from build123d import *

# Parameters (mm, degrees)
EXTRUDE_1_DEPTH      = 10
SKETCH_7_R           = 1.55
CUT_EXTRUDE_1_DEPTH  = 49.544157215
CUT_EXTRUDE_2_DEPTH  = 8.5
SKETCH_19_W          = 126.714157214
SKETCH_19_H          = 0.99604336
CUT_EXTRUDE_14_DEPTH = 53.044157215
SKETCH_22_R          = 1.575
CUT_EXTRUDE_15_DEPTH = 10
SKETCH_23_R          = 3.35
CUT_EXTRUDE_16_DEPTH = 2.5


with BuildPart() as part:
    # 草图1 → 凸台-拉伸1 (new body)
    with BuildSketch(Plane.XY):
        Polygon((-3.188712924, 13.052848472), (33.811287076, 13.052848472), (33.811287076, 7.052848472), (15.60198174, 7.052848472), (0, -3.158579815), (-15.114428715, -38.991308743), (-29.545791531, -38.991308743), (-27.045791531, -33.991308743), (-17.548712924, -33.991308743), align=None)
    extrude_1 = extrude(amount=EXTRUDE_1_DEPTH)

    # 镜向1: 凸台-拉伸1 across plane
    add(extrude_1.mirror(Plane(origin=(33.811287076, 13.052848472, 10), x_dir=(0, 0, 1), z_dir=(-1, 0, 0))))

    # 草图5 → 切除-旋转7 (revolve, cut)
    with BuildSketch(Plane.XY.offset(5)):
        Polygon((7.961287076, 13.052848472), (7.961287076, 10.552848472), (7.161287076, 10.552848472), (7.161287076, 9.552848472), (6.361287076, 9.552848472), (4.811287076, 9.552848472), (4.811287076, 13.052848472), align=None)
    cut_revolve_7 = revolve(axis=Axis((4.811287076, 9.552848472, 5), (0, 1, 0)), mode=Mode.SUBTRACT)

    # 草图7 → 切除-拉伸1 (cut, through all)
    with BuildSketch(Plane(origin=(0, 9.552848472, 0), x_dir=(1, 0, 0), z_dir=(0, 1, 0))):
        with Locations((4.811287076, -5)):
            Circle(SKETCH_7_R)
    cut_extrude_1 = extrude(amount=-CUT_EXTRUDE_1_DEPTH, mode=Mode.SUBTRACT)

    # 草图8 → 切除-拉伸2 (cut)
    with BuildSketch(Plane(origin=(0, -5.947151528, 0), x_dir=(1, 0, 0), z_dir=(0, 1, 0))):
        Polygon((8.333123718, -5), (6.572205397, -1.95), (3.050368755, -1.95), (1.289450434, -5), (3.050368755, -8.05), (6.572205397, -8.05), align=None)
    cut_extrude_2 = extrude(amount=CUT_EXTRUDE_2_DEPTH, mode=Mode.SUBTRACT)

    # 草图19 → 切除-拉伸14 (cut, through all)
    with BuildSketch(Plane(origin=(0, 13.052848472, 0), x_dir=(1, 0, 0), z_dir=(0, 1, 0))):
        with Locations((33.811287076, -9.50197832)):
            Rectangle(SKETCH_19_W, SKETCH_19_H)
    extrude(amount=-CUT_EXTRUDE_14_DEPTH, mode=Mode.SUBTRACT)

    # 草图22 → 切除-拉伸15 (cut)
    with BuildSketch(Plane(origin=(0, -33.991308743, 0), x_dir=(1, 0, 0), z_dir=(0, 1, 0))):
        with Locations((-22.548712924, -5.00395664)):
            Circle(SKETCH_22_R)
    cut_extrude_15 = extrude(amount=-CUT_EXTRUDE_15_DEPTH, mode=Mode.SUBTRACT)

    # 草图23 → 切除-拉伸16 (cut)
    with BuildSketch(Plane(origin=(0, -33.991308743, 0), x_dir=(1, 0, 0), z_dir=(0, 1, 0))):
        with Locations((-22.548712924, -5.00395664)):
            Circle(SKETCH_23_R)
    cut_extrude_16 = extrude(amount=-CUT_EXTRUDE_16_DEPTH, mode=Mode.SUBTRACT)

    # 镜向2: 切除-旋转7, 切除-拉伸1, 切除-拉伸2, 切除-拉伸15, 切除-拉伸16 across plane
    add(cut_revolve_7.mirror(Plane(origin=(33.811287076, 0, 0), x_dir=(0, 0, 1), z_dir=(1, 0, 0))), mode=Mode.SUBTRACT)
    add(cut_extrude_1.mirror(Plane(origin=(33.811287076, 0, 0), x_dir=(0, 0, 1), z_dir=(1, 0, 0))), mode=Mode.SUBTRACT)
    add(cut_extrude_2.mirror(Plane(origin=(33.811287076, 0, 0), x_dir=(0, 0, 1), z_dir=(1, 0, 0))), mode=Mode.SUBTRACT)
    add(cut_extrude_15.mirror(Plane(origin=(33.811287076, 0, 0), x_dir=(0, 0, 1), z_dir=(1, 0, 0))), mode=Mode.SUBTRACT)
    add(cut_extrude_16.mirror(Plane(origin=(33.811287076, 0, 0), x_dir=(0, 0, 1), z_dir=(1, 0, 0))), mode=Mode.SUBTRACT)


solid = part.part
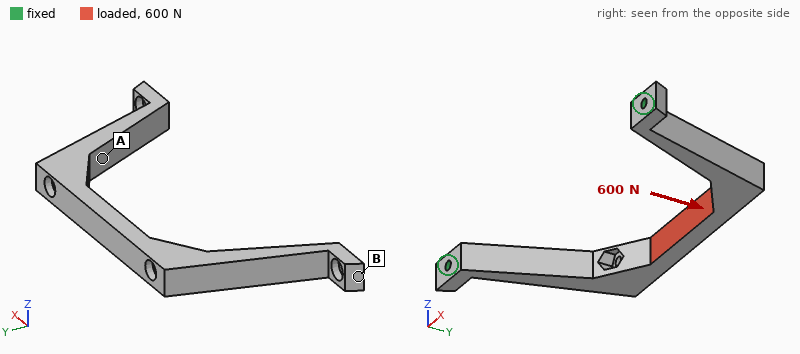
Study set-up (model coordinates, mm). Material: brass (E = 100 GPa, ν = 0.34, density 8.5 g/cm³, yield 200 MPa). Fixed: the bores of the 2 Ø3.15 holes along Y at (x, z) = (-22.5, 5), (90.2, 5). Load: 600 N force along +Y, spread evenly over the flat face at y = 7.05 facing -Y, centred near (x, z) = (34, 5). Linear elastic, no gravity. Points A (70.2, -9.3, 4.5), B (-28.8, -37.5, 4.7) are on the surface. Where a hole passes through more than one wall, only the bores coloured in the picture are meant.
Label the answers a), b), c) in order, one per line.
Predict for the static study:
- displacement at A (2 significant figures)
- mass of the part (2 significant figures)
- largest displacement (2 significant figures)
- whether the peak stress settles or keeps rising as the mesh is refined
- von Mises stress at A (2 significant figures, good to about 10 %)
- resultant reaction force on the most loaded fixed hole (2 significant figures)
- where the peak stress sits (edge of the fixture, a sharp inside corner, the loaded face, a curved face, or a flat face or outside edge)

a) 19 µm
b) 92 g
c) 54 µm
d) keeps rising
e) 37 MPa
f) 380 N
g) edge of the fixture
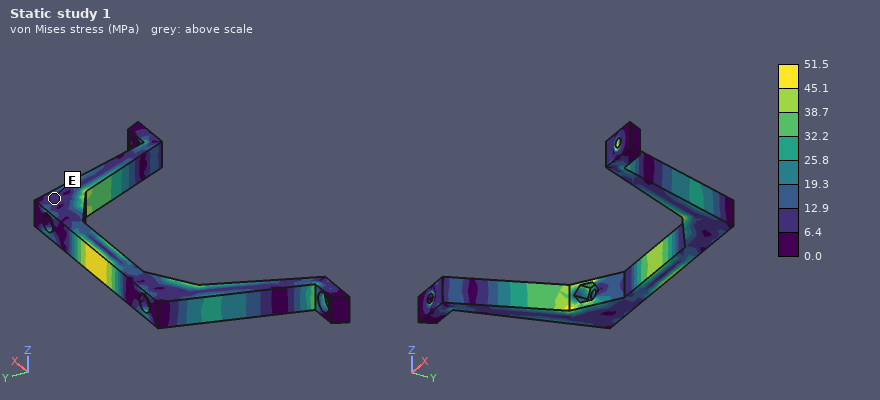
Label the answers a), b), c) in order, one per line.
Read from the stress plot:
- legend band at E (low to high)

a) 6.4 to 12.9 MPa
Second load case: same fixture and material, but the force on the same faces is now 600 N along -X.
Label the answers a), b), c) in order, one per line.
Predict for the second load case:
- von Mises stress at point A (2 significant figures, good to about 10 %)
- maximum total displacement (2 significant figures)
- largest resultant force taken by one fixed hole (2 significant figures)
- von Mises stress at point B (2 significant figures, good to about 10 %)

a) 56 MPa
b) 0.15 mm
c) 370 N
d) 11 MPa
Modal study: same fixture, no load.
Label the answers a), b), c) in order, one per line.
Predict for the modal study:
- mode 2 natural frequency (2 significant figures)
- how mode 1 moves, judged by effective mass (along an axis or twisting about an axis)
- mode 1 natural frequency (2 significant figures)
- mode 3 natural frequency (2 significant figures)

a) 1200 Hz
b) along Z
c) 490 Hz
d) 1300 Hz
